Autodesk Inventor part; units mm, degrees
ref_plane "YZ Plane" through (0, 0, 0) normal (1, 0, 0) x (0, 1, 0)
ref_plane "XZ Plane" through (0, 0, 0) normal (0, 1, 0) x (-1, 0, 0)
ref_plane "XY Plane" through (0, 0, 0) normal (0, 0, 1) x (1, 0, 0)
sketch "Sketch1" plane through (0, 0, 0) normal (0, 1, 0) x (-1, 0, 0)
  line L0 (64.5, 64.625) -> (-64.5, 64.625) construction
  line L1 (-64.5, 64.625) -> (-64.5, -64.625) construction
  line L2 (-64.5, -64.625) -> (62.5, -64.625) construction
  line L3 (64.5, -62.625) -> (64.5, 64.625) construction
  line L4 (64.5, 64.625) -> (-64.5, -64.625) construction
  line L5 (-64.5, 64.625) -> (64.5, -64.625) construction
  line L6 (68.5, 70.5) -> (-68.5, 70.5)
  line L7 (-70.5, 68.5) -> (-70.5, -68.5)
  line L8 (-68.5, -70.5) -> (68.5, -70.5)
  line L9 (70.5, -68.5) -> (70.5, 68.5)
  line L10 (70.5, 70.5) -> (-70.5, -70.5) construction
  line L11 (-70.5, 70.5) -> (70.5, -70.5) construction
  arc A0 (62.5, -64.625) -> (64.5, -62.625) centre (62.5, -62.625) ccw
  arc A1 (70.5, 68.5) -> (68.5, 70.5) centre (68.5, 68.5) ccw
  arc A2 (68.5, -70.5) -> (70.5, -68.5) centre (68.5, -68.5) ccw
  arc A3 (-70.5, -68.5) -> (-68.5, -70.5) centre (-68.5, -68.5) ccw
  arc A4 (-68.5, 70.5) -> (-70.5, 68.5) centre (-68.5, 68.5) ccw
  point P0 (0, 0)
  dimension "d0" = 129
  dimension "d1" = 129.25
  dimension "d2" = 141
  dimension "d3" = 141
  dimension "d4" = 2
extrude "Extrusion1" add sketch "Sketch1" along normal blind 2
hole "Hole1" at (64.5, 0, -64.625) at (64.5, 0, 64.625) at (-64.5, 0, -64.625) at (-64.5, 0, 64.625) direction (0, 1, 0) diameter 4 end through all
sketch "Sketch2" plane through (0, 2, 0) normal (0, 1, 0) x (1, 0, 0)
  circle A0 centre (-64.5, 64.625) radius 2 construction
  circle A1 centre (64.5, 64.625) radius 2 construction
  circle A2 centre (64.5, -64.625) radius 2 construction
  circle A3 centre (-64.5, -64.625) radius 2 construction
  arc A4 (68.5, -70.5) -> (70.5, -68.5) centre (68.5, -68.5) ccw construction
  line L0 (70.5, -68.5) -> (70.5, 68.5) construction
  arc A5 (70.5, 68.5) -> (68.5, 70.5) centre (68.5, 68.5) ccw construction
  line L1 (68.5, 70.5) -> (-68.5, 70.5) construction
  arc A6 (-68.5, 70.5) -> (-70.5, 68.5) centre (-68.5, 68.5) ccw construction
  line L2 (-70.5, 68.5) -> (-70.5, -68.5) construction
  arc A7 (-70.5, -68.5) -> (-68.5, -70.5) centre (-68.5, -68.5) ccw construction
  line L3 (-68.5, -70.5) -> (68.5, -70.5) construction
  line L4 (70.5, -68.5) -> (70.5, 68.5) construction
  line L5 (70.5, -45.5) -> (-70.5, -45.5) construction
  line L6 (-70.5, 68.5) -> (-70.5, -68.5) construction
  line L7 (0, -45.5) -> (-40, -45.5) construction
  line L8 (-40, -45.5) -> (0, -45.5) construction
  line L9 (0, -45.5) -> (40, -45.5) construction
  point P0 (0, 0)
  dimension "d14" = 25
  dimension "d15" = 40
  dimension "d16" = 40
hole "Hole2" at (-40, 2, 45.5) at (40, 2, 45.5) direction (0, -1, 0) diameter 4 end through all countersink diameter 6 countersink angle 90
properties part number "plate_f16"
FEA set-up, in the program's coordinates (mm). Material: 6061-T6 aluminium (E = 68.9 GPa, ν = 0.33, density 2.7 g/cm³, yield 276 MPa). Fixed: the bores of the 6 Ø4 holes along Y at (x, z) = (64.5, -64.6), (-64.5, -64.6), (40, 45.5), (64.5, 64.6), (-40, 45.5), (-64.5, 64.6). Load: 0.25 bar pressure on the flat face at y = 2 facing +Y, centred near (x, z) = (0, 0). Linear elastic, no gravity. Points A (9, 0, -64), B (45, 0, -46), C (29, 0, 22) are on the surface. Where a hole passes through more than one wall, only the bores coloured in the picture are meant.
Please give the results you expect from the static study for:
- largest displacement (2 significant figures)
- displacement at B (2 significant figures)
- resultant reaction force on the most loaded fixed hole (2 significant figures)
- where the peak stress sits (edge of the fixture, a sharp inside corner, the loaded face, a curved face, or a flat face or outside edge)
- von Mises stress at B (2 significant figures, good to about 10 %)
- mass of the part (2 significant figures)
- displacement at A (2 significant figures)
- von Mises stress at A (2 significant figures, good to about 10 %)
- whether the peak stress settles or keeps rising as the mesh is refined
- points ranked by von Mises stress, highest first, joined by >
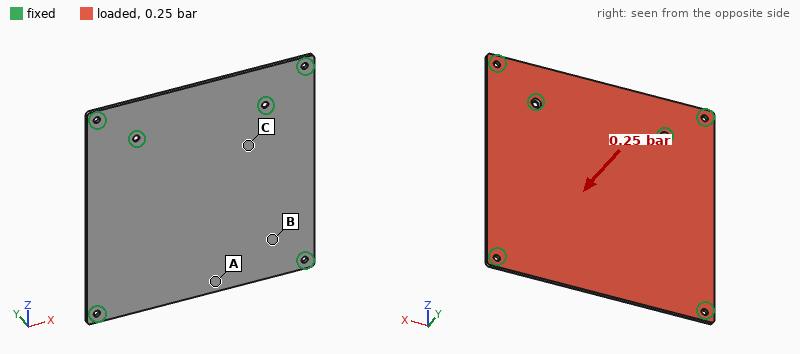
0.60 mm
0.28 mm
180 N
edge of the fixture
15 MPa
110 g
0.52 mm
31 MPa
keeps rising
A > B > C
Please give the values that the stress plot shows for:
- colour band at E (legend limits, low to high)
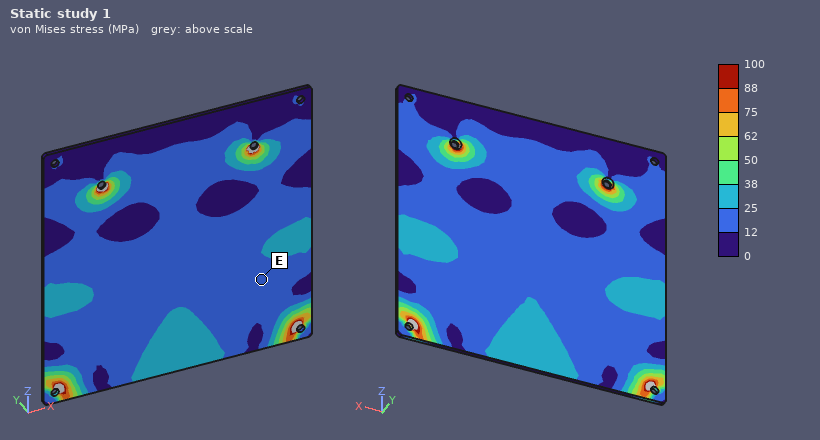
12 to 25 MPa
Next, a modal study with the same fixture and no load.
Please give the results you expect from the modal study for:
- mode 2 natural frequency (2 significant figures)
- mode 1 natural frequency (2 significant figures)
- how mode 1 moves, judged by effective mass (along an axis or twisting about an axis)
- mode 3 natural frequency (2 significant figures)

830 Hz
520 Hz
along Y
830 Hz
